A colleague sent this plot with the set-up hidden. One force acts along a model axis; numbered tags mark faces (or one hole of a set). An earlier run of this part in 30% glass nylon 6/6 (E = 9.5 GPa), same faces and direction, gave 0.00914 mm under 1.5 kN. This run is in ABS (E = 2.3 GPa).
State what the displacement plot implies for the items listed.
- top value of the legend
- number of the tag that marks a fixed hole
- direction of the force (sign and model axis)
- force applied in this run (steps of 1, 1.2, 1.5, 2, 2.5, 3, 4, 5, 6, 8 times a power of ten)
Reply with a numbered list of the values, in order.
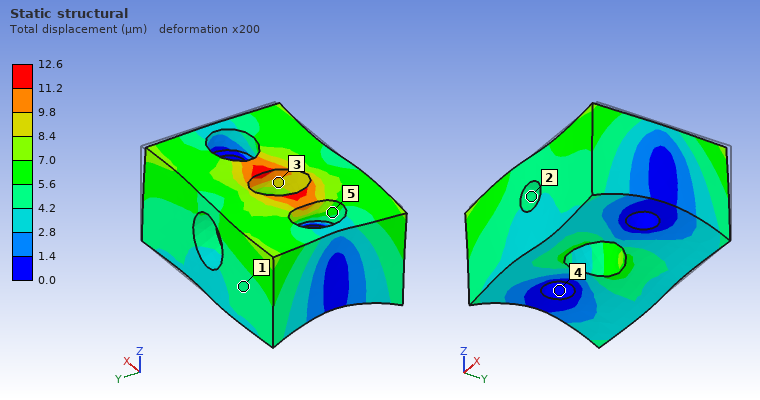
1. 12.6 µm
2. 4
3. -X
4. 500 N
